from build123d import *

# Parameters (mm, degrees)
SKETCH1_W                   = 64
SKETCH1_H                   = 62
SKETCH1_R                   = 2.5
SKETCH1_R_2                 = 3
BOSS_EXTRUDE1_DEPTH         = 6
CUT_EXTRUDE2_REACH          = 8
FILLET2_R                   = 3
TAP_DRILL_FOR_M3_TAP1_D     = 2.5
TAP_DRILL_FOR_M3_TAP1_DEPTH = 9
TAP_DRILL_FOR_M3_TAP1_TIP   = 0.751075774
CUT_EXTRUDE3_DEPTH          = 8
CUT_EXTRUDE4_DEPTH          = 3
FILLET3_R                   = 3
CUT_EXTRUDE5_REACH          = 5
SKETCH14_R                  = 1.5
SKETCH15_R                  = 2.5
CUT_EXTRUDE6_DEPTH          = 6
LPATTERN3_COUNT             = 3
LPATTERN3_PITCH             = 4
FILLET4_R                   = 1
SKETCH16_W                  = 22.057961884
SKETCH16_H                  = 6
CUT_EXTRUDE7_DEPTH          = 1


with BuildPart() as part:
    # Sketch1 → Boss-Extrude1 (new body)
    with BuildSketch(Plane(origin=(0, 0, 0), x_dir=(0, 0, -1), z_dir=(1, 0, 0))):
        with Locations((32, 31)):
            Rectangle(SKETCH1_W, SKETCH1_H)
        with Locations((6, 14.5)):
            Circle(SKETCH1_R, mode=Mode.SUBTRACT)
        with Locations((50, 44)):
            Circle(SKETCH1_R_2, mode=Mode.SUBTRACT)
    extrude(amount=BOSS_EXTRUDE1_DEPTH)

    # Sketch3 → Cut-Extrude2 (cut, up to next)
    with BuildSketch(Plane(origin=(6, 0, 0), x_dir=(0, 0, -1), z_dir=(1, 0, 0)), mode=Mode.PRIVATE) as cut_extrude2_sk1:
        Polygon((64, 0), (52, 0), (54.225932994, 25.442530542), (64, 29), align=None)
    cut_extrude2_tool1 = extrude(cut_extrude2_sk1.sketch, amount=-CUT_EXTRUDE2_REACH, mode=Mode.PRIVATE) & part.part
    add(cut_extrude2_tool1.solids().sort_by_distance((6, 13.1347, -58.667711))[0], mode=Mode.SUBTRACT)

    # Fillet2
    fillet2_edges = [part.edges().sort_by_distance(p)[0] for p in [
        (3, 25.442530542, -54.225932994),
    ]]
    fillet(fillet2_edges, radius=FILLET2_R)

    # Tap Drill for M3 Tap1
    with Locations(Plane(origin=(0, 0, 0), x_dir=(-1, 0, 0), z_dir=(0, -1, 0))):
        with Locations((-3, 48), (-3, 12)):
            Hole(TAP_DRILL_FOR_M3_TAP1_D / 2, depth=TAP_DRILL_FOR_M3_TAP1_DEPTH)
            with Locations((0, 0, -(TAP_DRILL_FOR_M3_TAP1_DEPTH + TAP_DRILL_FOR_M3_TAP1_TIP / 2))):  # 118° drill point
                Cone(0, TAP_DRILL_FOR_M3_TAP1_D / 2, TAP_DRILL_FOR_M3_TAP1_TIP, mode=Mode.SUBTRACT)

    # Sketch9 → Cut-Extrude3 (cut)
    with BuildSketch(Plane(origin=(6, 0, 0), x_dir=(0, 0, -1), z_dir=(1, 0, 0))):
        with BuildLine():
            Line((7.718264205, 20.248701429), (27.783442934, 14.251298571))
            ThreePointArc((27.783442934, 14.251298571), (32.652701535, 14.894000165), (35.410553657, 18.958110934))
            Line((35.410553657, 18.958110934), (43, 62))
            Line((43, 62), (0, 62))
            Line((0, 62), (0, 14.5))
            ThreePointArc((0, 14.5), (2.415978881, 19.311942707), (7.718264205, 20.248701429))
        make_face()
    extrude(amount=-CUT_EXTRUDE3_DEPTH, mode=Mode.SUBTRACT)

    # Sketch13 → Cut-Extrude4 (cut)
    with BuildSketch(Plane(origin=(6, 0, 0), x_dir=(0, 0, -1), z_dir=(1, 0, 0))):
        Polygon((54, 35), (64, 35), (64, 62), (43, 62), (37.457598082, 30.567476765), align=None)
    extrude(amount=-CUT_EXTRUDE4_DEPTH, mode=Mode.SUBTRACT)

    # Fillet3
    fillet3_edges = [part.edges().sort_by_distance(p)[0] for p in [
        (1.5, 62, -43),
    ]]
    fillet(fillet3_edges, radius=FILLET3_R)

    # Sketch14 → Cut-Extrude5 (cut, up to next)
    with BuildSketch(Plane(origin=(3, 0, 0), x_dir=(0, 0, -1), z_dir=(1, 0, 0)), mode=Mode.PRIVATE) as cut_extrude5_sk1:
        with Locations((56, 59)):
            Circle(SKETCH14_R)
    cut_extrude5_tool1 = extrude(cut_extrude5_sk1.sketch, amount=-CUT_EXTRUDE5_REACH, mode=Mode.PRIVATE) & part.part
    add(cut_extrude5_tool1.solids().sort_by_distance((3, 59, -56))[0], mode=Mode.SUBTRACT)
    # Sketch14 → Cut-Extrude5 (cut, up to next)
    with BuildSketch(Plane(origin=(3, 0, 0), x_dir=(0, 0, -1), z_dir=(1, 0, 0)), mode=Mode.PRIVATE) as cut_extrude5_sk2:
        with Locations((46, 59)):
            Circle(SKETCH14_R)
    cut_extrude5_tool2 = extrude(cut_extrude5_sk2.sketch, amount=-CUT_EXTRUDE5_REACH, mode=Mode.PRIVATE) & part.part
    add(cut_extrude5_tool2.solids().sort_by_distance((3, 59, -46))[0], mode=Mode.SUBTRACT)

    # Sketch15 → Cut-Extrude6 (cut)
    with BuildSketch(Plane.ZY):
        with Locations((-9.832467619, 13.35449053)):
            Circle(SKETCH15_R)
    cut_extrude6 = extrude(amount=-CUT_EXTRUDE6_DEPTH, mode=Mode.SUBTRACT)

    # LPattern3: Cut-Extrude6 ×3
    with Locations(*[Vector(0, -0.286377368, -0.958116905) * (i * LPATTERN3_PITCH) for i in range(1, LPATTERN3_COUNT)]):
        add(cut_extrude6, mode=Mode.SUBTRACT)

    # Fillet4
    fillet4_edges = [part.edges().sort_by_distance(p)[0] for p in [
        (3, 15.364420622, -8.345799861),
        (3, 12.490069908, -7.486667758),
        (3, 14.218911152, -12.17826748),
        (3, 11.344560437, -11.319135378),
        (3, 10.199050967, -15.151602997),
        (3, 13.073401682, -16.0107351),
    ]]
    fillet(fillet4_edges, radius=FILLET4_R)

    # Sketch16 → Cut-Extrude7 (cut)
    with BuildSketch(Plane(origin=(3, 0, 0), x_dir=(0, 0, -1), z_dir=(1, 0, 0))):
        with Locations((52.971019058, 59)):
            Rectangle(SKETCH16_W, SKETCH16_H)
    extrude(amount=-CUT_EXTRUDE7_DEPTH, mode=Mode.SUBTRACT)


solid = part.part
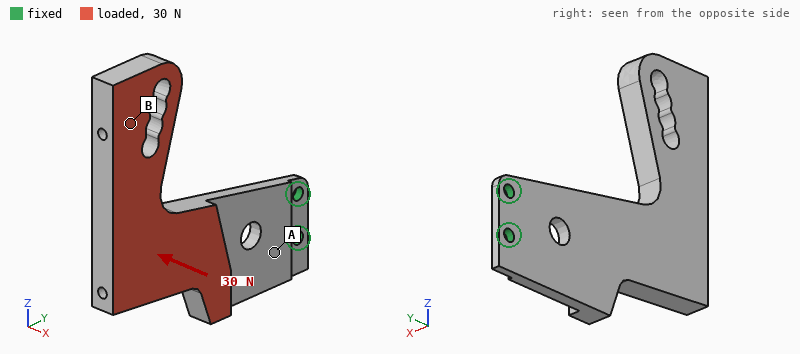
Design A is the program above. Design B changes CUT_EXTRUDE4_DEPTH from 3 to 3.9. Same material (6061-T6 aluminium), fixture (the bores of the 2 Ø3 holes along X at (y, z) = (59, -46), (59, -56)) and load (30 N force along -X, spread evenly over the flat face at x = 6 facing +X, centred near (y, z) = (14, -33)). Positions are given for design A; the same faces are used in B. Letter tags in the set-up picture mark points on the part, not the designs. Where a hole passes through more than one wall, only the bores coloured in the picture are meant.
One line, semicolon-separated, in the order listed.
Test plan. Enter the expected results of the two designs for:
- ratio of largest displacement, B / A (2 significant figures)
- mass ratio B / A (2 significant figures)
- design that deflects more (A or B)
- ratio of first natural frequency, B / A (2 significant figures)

2.0; 0.95; B; 0.71
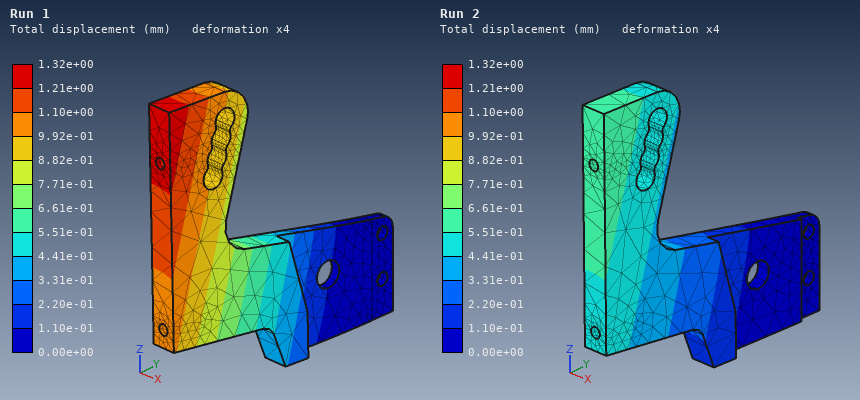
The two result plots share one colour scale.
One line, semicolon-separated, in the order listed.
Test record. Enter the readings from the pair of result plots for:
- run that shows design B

Run 1
